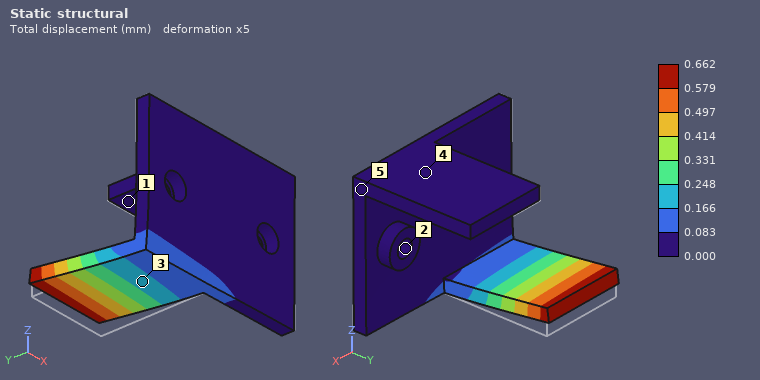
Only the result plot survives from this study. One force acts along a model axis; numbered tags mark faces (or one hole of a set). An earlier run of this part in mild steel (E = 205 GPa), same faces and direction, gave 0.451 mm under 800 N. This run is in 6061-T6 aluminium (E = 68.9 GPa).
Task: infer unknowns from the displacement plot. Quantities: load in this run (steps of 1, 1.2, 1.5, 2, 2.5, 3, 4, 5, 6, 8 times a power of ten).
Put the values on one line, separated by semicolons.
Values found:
400 N
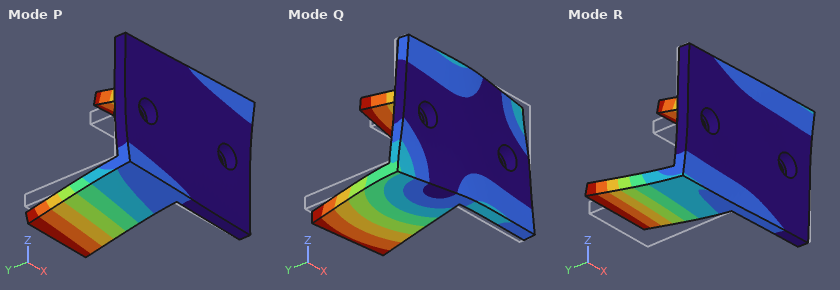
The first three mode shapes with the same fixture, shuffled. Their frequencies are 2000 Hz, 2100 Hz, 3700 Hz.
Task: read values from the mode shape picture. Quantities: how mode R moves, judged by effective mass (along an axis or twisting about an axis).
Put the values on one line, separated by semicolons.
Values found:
along Z
